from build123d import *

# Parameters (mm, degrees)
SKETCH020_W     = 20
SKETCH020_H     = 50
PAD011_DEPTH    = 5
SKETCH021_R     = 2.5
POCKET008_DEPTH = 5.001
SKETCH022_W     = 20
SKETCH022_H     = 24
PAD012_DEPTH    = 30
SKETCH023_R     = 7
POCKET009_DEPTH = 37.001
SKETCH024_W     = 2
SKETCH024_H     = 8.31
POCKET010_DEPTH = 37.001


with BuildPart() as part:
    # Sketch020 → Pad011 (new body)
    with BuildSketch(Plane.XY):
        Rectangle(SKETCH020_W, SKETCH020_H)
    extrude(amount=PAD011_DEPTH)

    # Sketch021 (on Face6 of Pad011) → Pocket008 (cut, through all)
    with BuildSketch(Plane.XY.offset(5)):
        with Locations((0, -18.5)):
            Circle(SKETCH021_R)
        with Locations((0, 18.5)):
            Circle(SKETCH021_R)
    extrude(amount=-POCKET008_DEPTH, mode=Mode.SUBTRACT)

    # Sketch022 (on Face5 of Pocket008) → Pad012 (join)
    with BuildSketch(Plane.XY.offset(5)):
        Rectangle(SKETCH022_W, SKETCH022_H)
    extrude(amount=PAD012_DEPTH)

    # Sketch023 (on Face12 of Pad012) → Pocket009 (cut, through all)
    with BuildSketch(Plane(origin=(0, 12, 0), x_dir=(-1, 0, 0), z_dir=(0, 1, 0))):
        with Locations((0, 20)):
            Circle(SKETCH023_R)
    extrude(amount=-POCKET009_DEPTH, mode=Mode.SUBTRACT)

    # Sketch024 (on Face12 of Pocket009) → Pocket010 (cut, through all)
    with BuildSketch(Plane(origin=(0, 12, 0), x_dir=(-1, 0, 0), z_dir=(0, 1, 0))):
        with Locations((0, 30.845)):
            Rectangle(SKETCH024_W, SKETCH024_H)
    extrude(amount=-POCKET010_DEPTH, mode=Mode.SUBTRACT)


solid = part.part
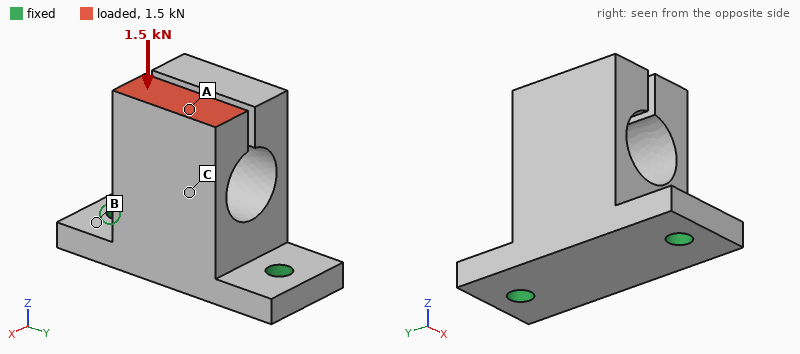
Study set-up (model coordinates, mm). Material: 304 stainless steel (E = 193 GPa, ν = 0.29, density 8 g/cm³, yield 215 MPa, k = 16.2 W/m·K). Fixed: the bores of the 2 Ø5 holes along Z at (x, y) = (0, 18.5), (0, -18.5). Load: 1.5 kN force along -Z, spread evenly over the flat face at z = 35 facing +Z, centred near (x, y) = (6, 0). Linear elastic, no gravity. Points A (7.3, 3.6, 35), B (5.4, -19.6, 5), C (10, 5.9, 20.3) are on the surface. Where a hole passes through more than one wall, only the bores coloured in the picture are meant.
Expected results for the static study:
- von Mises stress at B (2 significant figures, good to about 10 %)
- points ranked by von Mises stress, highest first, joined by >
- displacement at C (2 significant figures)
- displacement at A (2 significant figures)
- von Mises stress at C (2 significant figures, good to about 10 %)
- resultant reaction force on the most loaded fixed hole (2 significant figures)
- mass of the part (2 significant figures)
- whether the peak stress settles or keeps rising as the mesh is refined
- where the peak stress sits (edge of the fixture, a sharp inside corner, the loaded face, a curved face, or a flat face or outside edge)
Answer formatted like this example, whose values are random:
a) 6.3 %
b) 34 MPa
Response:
a) 26 MPa
b) C > B > A
c) 6.7 µm
d) 31 µm
e) 84 MPa
f) 810 N
g) 120 g
h) keeps rising
i) edge of the fixture
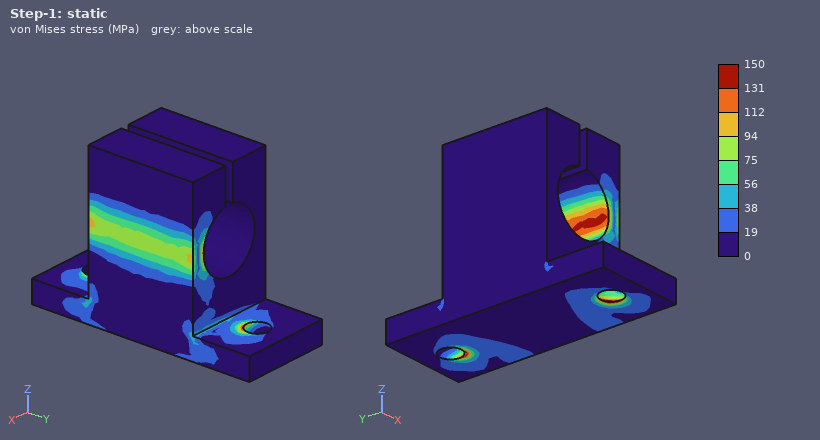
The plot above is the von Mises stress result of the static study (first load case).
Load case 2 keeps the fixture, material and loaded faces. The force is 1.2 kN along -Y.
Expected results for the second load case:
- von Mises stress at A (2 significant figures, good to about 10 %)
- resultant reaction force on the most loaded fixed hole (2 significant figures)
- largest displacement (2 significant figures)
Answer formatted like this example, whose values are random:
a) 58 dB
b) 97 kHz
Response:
a) 11 MPa
b) 1.5 kN
c) 34 µm
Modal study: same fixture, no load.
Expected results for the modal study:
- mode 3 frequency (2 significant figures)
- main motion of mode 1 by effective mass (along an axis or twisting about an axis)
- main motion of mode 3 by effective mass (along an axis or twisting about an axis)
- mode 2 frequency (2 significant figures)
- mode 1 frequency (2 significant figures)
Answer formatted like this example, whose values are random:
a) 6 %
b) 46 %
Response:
a) 7600 Hz
b) along X
c) along Y
d) 3700 Hz
e) 2700 Hz
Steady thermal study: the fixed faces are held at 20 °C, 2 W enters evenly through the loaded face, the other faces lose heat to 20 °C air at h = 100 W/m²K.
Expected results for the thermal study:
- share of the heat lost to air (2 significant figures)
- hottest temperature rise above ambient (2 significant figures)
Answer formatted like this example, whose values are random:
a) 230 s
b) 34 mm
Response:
a) 82 %
b) 15 K
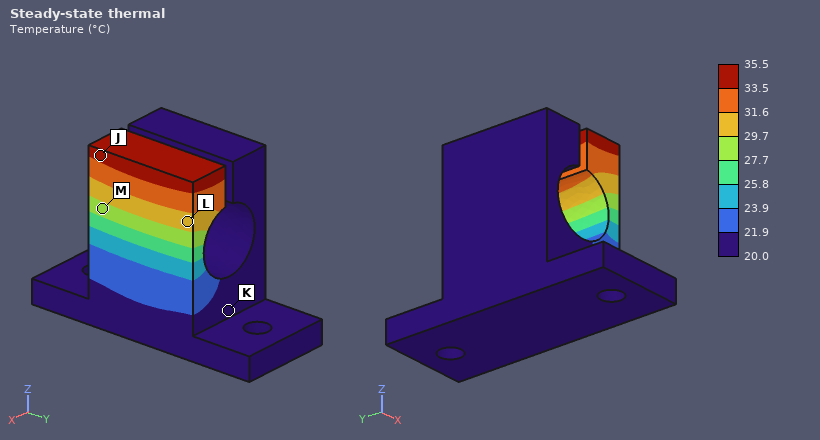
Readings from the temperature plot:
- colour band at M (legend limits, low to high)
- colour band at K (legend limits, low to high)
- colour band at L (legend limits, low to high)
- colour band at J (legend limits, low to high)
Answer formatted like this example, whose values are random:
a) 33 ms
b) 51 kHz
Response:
a) 27.7 to 29.7 °C
b) 20.0 to 21.9 °C
c) 29.7 to 31.6 °C
d) 33.5 to 35.5 °C
